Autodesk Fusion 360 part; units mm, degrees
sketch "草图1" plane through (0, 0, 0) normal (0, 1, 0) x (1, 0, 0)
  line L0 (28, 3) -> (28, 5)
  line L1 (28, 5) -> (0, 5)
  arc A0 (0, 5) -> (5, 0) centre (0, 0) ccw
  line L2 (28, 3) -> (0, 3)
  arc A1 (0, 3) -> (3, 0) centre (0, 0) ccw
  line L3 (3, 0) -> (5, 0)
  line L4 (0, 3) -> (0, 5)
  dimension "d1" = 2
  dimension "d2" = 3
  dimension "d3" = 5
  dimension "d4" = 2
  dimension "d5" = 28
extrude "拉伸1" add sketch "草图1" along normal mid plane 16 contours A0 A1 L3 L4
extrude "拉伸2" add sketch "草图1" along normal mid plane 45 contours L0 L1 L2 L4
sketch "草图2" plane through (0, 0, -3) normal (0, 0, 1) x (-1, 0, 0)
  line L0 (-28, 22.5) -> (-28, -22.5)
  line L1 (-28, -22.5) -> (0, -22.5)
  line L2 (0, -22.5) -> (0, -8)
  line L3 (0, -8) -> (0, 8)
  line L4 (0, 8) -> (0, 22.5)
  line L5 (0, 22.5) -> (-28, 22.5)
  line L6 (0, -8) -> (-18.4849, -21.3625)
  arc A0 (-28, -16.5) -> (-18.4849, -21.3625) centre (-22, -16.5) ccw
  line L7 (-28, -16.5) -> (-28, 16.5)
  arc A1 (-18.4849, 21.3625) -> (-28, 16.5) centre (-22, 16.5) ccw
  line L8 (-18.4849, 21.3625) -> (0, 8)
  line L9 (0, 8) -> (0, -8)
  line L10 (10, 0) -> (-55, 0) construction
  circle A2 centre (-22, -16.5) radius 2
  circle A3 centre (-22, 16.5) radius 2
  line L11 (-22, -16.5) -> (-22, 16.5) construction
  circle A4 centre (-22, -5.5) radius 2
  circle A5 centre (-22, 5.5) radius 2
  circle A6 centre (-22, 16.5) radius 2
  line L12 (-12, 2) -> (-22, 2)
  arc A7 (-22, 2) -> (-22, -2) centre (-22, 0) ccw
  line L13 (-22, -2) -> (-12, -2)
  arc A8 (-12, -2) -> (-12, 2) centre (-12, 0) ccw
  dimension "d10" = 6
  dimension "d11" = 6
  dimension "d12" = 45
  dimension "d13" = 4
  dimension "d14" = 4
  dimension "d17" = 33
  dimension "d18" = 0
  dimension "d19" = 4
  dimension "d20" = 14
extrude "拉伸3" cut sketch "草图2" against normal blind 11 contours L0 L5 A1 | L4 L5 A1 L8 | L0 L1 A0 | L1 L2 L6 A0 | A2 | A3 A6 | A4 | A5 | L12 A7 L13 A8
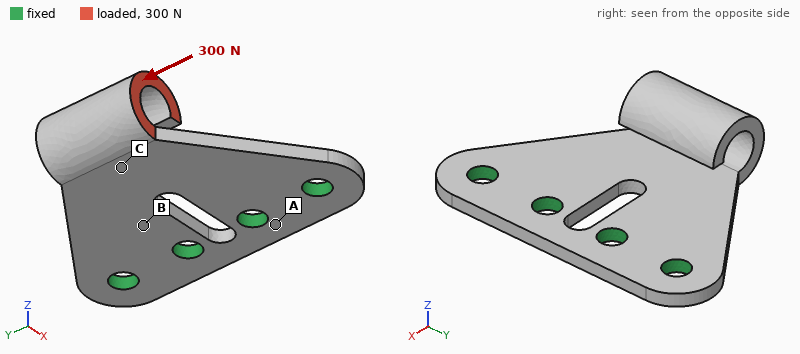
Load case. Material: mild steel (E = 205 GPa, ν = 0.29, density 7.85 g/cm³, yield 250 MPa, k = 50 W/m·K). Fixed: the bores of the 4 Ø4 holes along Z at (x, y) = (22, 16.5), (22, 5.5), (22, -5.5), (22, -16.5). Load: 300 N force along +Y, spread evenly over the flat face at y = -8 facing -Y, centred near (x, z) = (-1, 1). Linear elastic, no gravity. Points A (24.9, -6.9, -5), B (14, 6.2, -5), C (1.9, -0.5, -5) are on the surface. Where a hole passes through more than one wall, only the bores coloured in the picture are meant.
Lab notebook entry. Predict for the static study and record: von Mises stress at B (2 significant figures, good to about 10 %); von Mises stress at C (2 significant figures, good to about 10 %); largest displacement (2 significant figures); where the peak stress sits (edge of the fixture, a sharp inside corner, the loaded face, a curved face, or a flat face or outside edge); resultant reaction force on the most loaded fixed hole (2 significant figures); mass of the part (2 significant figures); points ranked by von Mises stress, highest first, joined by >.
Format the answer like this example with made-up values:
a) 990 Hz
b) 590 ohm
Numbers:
a) 35 MPa
b) 69 MPa
c) 71 µm
d) a curved face
e) 210 N
f) 18 g
g) C > B > A
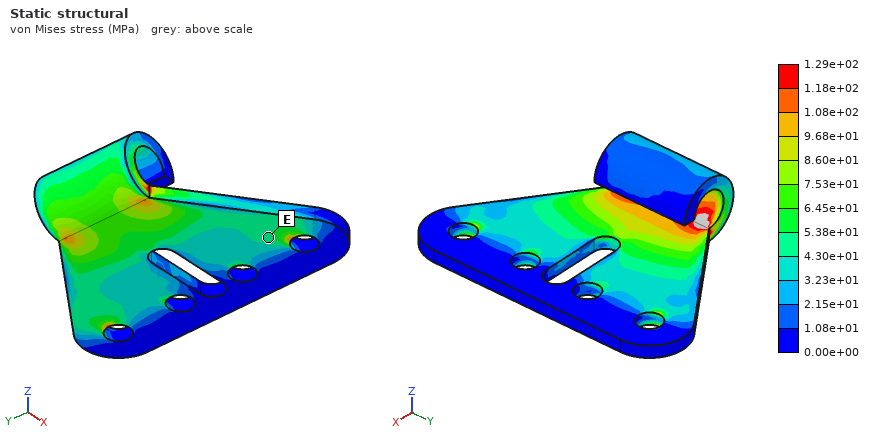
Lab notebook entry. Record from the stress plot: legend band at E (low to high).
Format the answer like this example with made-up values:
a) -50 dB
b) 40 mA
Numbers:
a) 4.30e+01 to 5.38e+01 MPa
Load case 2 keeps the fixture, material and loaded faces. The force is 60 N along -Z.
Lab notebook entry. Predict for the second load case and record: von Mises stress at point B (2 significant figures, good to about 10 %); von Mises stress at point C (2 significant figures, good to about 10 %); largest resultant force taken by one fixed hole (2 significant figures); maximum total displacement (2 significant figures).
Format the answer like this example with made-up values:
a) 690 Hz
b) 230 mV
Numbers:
a) 40 MPa
b) 29 MPa
c) 25 N
d) 80 µm
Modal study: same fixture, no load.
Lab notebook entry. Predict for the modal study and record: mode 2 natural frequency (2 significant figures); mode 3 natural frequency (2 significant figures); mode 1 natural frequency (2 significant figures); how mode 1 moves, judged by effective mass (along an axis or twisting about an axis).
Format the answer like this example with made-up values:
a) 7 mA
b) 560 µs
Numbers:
a) 4800 Hz
b) 5800 Hz
c) 2100 Hz
d) along Z
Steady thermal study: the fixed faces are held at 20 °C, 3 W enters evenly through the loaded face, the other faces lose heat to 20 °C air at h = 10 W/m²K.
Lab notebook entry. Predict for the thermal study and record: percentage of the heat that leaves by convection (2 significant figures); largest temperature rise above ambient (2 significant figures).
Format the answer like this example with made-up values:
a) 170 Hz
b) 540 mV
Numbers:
a) 12 %
b) 48 K
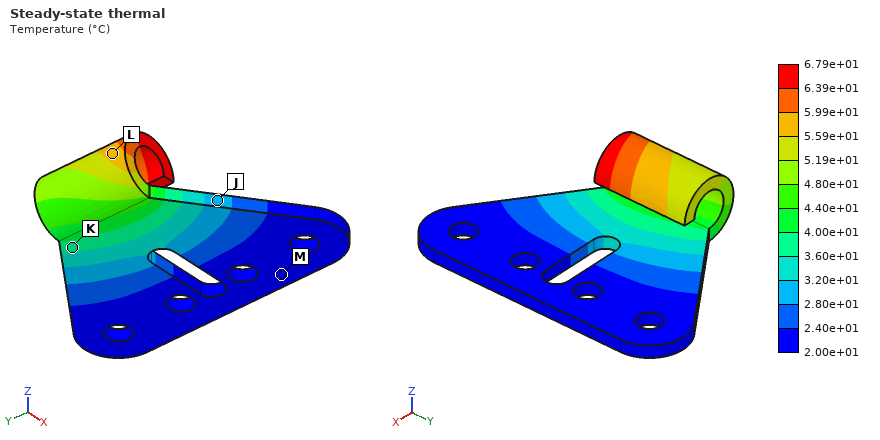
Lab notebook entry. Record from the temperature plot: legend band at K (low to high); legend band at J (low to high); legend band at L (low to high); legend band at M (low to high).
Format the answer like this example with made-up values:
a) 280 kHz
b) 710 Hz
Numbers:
a) 3.60e+01 to 4.00e+01 °C
b) 2.80e+01 to 3.20e+01 °C
c) 5.59e+01 to 5.99e+01 °C
d) 2.00e+01 to 2.40e+01 °C
